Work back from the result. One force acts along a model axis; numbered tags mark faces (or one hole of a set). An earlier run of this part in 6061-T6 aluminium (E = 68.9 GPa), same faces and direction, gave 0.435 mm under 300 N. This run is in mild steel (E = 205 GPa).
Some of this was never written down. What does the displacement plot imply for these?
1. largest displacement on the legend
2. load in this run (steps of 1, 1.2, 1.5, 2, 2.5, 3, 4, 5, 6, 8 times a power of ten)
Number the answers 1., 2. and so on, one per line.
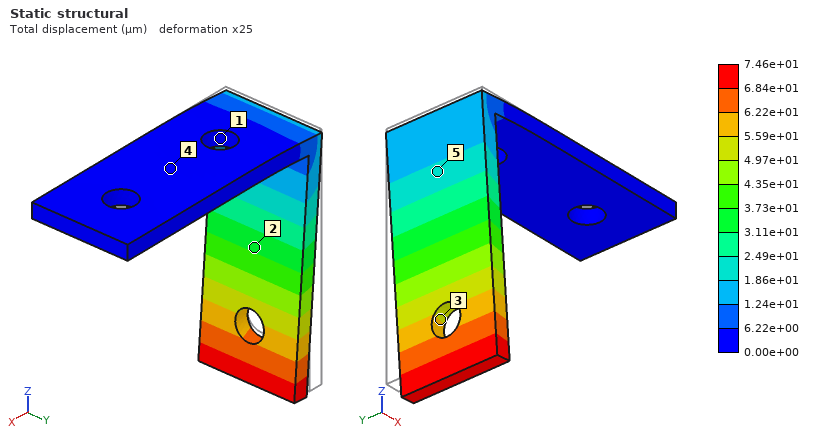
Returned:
1. 7.46e+01 µm
2. 150 N
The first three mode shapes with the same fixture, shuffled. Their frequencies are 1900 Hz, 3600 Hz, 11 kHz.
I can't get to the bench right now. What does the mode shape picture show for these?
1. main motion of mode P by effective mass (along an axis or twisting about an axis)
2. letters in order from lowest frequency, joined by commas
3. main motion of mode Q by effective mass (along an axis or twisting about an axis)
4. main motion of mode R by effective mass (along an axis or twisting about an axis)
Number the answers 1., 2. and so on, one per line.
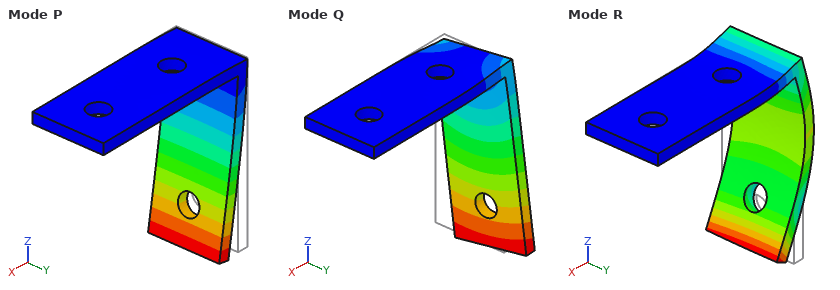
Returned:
1. along X
2. P, Q, R
3. along Y
4. along Z
